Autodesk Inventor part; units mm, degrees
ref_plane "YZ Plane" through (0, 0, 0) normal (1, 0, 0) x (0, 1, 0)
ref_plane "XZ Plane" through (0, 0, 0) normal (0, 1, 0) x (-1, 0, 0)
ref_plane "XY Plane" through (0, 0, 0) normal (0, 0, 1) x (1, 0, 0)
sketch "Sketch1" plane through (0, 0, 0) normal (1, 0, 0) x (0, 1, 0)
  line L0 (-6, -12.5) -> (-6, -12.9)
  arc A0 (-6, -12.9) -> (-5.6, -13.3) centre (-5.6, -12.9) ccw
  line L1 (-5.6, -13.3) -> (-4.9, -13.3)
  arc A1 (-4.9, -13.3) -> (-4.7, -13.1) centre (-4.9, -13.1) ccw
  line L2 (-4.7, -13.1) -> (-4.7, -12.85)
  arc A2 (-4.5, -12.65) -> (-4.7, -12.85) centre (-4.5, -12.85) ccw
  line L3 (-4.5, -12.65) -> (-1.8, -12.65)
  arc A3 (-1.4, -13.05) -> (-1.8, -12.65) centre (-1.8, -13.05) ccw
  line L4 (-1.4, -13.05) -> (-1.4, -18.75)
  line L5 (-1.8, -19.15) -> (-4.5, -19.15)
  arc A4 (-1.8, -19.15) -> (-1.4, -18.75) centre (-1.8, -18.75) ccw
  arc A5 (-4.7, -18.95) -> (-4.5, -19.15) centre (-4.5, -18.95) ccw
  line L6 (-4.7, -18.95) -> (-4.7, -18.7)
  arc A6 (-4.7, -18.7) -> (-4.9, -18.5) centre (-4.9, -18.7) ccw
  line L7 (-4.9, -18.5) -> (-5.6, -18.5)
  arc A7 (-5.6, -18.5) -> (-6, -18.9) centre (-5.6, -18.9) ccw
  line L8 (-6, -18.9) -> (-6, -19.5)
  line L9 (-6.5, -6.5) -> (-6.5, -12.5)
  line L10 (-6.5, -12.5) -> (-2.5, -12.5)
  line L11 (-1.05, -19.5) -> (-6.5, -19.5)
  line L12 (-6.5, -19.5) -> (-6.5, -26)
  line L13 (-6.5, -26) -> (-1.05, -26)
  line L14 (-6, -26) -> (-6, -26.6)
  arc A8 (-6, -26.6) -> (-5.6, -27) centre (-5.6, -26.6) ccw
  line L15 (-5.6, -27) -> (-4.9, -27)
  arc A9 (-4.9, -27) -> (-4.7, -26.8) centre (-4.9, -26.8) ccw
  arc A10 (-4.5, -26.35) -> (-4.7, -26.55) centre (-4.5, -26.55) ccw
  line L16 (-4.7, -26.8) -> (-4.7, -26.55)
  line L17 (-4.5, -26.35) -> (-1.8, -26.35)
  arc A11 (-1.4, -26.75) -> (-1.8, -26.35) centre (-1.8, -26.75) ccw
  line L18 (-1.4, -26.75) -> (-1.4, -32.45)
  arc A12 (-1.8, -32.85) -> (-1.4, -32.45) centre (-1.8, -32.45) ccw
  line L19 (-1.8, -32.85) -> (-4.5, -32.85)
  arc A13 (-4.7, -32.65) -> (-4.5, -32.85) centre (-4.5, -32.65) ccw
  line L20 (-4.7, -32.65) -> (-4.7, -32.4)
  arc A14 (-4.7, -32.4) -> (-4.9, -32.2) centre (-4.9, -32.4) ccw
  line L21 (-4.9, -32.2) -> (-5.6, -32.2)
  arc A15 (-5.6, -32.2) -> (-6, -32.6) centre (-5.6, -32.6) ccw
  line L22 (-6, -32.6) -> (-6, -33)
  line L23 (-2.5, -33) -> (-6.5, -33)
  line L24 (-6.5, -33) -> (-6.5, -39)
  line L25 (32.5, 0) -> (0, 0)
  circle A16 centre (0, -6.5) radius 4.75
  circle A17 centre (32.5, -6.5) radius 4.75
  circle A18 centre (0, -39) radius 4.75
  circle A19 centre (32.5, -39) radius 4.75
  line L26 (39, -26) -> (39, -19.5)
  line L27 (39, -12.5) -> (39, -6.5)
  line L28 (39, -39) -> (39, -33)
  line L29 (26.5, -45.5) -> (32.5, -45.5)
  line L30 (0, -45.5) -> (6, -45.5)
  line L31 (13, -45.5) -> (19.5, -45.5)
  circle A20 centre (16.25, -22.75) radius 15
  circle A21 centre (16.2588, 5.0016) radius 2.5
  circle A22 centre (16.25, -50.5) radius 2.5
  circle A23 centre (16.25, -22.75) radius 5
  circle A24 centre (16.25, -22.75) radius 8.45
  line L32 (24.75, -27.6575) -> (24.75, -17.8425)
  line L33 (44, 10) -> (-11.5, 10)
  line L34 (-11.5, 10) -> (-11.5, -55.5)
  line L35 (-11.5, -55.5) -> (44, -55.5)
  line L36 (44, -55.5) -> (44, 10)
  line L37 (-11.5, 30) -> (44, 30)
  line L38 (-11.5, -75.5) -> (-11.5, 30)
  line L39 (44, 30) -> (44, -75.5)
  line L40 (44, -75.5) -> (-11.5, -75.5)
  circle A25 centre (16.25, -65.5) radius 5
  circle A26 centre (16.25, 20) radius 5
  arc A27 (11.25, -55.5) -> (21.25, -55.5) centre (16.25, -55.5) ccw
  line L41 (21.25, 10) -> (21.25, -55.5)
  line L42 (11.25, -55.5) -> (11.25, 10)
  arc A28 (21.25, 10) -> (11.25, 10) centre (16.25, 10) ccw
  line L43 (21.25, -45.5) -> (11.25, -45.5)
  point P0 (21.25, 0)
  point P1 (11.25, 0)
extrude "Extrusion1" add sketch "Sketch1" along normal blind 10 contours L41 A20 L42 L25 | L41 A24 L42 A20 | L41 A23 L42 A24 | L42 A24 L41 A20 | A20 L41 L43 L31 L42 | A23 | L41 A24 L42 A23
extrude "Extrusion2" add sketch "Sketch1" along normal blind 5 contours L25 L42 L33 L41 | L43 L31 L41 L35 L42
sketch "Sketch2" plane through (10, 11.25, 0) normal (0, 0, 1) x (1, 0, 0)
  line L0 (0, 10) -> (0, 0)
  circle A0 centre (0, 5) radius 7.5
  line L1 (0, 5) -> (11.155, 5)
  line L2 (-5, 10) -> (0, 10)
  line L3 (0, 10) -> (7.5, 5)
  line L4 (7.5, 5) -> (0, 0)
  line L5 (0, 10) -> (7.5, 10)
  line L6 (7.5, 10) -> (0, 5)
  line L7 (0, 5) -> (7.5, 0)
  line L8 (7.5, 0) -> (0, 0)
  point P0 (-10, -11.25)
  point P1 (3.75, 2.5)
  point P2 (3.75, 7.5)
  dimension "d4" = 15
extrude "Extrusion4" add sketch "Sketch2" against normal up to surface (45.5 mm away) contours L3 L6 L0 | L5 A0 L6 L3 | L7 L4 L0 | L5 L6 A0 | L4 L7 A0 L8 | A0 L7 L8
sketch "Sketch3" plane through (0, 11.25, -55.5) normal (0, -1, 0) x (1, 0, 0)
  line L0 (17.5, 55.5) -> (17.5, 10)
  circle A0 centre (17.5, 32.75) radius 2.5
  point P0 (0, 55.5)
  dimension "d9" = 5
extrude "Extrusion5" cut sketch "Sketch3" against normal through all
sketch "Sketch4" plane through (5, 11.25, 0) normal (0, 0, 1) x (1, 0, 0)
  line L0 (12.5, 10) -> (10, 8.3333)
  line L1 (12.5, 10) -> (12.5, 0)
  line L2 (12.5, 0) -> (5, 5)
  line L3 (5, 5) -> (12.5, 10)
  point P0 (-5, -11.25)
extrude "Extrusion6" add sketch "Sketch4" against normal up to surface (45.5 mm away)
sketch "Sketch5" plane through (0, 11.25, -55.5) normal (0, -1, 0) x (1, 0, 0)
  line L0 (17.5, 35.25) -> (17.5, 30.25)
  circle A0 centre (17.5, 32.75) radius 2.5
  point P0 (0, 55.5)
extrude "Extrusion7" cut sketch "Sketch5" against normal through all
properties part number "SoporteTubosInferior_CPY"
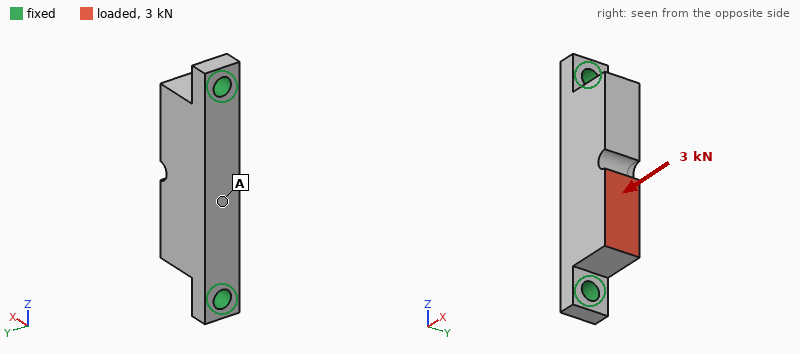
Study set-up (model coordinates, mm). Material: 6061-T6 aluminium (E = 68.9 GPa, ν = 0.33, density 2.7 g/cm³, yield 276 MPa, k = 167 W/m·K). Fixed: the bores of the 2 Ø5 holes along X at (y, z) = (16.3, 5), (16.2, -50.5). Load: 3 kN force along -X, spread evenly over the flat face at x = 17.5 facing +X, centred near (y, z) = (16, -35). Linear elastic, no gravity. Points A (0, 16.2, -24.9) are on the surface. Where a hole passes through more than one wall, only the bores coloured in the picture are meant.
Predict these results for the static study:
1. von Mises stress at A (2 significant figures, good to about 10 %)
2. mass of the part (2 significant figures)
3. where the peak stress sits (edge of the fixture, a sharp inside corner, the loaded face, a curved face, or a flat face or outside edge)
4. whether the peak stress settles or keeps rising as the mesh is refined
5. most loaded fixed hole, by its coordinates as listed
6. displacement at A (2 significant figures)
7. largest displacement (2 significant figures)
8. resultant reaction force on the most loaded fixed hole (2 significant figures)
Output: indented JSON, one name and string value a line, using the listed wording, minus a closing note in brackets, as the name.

{
  "von Mises stress at A": "21 MPa",
  "mass of the part": "23 g",
  "where the peak stress sits": "edge of the fixture",
  "whether the peak stress settles or keeps rising as the mesh is refined": "keeps rising",
  "most loaded fixed hole, by its coordinates as listed": "(16.2, -50.5)",
  "displacement at A": "23 µm",
  "largest displacement": "24 µm",
  "resultant reaction force on the most loaded fixed hole": "2.5 kN"
}
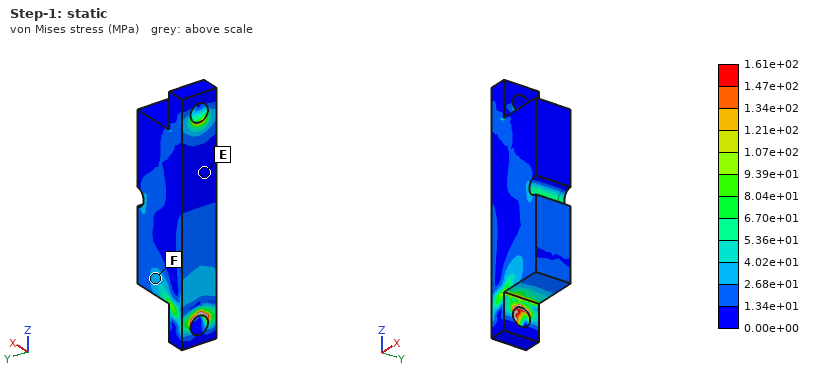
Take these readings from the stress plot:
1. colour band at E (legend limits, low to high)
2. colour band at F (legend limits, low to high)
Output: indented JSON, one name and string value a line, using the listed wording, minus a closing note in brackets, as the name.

{
  "colour band at E": "0.00e+00 to 1.34e+01 MPa",
  "colour band at F": "2.68e+01 to 4.02e+01 MPa"
}
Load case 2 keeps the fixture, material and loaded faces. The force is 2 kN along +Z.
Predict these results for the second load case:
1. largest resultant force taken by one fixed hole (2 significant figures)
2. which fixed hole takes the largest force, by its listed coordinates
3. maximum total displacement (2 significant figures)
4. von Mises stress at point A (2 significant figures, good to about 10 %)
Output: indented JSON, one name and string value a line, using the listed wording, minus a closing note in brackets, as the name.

{
  "largest resultant force taken by one fixed hole": "1.3 kN",
  "which fixed hole takes the largest force, by its listed coordinates": "(16.3, 5)",
  "maximum total displacement": "15 µm",
  "von Mises stress at point A": "13 MPa"
}
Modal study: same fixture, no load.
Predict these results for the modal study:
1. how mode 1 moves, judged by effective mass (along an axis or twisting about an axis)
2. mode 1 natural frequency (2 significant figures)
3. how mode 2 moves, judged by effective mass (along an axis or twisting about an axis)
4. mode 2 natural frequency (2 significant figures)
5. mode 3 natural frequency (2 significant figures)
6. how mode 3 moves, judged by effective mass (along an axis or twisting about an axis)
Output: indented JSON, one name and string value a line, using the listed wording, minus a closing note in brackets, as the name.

{
  "how mode 1 moves, judged by effective mass": "along Y",
  "mode 1 natural frequency": "6600 Hz",
  "how mode 2 moves, judged by effective mass": "along X",
  "mode 2 natural frequency": "13 kHz",
  "mode 3 natural frequency": "15 kHz",
  "how mode 3 moves, judged by effective mass": "along Y"
}
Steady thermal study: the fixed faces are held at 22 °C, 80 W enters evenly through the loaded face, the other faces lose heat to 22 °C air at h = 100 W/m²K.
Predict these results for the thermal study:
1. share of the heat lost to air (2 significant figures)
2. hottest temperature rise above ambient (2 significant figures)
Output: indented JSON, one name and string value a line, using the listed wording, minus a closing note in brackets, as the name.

{
  "share of the heat lost to air": "12 %",
  "hottest temperature rise above ambient": "65 K"
}
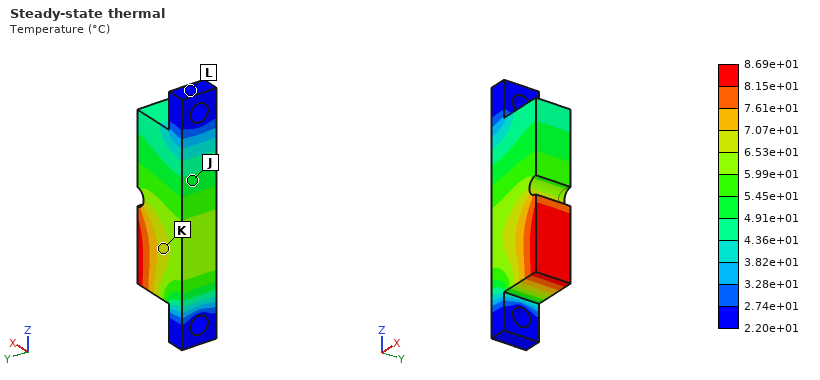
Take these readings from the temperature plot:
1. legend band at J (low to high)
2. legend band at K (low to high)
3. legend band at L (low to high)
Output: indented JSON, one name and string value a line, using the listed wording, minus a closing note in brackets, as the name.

{
  "legend band at J": "4.91e+01 to 5.45e+01 °C",
  "legend band at K": "6.53e+01 to 7.07e+01 °C",
  "legend band at L": "2.20e+01 to 2.74e+01 °C"
}
